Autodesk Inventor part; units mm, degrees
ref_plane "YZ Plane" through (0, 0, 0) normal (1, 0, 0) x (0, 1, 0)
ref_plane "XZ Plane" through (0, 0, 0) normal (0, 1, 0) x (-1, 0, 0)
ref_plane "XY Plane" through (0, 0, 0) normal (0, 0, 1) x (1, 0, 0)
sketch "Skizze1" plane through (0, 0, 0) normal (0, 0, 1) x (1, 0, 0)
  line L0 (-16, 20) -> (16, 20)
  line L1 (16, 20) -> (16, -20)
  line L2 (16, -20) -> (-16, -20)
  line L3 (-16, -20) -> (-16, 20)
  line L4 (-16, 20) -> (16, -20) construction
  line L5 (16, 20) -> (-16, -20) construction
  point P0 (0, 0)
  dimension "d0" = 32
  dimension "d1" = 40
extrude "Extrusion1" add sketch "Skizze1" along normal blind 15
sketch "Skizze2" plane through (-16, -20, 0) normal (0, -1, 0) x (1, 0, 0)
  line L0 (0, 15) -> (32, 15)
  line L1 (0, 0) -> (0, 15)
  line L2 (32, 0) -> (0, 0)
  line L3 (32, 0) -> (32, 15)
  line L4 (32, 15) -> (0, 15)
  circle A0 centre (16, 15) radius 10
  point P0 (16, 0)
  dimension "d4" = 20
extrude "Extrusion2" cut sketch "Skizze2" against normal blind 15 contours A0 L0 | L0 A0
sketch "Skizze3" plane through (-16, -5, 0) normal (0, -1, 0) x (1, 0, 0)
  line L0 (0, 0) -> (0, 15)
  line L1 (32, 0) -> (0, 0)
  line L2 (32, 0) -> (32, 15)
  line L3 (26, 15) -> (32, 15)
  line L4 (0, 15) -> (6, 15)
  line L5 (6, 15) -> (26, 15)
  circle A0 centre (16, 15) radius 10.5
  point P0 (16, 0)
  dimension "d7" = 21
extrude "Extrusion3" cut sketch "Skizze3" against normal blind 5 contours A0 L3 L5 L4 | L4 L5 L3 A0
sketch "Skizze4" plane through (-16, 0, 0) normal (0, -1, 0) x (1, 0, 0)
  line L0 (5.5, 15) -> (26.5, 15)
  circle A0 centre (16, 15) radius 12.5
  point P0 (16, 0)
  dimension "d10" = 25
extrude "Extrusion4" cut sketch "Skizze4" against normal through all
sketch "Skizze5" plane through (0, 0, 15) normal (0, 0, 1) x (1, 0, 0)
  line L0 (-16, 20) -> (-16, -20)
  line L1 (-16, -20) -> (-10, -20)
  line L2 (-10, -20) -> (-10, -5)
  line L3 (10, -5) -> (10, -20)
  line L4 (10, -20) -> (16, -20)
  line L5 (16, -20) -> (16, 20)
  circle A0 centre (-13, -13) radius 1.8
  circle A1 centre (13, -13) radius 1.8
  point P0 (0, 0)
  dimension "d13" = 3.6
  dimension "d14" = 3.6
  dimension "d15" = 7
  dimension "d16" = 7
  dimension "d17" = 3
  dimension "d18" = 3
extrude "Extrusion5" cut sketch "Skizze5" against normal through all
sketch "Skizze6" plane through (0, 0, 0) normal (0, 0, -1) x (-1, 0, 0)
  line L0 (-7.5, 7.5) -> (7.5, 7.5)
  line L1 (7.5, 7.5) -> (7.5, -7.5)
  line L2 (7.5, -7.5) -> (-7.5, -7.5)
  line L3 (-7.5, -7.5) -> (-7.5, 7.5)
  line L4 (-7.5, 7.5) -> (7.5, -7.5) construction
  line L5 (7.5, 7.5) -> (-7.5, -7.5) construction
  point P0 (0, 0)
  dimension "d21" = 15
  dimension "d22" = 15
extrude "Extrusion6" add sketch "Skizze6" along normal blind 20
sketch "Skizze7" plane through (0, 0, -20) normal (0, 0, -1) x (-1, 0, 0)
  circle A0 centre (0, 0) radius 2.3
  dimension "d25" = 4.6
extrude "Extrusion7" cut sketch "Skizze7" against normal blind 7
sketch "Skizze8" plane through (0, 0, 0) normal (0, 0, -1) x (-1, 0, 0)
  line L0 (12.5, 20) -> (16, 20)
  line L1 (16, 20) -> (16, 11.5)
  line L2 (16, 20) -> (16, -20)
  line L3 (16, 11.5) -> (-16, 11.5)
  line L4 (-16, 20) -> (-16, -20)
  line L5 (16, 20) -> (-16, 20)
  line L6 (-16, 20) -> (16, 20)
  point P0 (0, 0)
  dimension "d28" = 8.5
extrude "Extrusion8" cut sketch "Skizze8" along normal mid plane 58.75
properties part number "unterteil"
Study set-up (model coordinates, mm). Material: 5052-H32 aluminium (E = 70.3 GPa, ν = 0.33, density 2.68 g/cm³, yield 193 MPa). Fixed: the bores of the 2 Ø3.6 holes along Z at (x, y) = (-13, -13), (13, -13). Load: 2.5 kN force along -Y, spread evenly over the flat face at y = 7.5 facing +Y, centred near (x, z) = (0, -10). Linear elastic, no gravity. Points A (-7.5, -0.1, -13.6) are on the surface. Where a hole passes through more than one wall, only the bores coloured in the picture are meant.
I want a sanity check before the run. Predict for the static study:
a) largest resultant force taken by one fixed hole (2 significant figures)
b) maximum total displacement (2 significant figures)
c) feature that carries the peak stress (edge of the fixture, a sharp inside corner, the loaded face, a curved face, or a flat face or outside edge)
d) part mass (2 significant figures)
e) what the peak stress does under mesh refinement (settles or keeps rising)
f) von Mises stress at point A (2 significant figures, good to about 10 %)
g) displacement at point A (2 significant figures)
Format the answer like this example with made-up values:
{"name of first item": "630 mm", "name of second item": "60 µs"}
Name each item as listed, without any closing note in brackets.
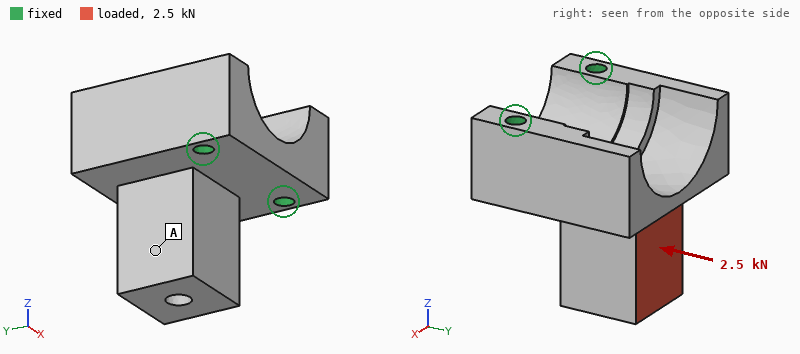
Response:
{"largest resultant force taken by one fixed hole": "1.4 kN", "maximum total displacement": "89 µm", "feature that carries the peak stress": "edge of the fixture", "part mass": "35 g", "what the peak stress does under mesh refinement": "keeps rising", "von Mises stress at point A": "12 MPa", "displacement at point A": "60 µm"}
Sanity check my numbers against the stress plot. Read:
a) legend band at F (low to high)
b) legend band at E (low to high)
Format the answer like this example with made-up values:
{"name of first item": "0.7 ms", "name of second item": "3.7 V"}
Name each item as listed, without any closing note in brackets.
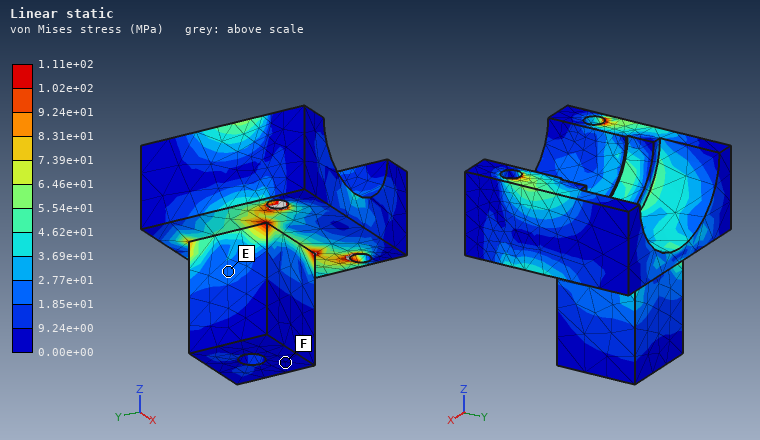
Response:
{"legend band at F": "0.00e+00 to 9.24e+00 MPa", "legend band at E": "1.85e+01 to 2.77e+01 MPa"}
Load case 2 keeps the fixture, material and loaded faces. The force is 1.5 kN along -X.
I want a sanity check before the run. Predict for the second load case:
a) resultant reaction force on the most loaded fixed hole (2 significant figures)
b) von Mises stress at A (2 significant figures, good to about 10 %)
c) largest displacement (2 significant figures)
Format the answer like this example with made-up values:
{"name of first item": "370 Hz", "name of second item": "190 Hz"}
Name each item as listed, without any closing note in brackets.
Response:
{"resultant reaction force on the most loaded fixed hole": "1.7 kN", "von Mises stress at A": "10 MPa", "largest displacement": "33 µm"}
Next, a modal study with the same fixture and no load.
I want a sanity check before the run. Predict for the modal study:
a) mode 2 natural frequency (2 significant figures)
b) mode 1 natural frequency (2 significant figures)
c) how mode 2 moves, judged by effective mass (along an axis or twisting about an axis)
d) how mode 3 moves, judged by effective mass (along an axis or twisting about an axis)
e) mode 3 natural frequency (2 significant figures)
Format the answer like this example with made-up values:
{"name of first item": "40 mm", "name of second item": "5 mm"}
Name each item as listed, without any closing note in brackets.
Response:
{"mode 2 natural frequency": "12 kHz", "mode 1 natural frequency": "8400 Hz", "how mode 2 moves, judged by effective mass": "along X", "how mode 3 moves, judged by effective mass": "along X", "mode 3 natural frequency": "18 kHz"}
